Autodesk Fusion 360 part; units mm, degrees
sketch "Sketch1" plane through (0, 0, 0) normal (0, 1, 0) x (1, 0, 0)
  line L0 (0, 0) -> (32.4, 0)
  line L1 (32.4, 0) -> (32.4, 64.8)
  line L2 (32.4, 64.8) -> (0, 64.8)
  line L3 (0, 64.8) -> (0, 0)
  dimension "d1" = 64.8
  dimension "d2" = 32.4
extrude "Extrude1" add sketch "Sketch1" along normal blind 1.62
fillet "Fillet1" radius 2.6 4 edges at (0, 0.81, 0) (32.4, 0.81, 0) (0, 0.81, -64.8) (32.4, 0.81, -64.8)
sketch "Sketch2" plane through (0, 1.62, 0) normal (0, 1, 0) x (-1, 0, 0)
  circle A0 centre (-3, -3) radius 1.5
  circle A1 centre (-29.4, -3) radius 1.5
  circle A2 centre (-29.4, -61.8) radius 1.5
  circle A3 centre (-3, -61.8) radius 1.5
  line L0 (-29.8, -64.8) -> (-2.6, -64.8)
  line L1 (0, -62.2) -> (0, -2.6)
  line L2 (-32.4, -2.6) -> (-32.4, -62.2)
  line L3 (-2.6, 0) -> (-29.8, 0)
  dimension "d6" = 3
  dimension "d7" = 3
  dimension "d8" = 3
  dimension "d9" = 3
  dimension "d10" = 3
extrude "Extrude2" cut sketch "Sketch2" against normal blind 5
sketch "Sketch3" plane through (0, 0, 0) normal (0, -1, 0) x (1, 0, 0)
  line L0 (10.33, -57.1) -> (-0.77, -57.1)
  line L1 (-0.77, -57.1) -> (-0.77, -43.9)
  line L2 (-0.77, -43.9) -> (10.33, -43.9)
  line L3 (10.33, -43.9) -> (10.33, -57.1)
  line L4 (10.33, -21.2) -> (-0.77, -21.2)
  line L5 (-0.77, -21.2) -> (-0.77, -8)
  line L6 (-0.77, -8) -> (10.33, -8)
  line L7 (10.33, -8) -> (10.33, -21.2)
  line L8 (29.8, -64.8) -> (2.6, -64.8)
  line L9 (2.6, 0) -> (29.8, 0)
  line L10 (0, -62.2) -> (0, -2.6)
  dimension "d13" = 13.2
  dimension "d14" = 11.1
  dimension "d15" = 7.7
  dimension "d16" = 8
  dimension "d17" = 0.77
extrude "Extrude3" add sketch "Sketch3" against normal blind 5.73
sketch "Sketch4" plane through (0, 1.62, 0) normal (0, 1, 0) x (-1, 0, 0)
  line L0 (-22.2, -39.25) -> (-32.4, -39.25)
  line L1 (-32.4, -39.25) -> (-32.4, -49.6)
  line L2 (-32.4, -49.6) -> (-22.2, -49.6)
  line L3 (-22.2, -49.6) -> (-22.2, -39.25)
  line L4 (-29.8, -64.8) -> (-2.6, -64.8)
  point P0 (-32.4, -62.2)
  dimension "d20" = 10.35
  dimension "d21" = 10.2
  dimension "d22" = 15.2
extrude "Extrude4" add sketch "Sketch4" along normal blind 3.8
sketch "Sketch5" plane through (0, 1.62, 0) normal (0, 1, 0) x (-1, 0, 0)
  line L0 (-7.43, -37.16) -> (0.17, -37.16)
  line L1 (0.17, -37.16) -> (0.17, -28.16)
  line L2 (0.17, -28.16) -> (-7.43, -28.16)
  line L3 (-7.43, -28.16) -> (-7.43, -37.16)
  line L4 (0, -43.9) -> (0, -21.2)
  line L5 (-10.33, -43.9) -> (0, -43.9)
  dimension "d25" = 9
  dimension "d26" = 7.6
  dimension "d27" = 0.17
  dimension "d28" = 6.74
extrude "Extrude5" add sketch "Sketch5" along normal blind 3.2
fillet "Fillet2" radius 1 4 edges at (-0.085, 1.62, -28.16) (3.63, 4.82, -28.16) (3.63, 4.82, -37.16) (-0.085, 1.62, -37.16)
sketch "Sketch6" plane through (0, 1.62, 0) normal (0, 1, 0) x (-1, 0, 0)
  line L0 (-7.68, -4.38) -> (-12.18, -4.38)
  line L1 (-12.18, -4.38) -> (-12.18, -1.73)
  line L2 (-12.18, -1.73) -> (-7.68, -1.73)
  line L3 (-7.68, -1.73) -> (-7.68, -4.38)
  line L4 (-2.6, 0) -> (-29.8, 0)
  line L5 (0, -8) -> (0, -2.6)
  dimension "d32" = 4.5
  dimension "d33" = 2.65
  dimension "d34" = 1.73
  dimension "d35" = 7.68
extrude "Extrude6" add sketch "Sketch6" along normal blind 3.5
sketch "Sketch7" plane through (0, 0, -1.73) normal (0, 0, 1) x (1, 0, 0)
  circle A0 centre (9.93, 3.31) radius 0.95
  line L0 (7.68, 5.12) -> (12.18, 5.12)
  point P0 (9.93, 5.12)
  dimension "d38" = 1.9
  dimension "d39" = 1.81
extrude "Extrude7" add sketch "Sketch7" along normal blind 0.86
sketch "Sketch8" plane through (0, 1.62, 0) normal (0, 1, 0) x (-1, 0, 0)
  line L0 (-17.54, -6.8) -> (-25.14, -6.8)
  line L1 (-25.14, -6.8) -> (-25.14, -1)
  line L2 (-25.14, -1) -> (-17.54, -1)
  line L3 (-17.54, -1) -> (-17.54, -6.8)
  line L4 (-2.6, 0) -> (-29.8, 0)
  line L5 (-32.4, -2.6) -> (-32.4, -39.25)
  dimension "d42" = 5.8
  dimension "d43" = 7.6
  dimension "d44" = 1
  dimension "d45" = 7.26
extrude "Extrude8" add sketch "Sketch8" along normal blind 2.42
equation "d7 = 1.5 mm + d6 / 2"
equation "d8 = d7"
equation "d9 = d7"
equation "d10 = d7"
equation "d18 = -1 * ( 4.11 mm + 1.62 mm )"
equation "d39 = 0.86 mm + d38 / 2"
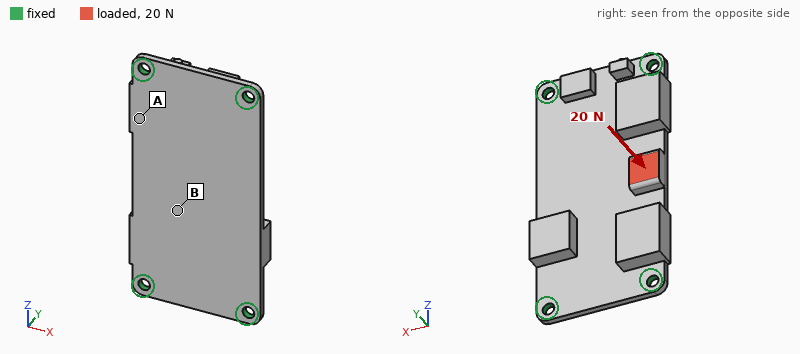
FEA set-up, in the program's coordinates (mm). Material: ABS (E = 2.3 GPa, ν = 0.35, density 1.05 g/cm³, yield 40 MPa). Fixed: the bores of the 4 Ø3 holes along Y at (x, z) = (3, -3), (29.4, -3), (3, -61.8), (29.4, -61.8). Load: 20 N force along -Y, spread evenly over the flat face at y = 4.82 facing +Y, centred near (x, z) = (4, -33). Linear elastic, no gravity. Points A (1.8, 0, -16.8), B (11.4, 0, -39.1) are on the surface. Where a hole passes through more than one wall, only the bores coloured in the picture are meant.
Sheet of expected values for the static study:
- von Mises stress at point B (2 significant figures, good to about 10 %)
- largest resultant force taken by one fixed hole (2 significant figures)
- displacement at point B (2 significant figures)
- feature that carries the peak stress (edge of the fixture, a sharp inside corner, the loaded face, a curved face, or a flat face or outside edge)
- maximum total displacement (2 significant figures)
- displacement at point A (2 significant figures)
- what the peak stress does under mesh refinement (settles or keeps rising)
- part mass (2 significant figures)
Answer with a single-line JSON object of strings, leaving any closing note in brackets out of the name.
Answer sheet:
{"von Mises stress at point B": "5.4 MPa", "largest resultant force taken by one fixed hole": "9.4 N", "displacement at point B": "0.60 mm", "feature that carries the peak stress": "edge of the fixture", "maximum total displacement": "0.81 mm", "displacement at point A": "0.40 mm", "what the peak stress does under mesh refinement": "keeps rising", "part mass": "5.6 g"}
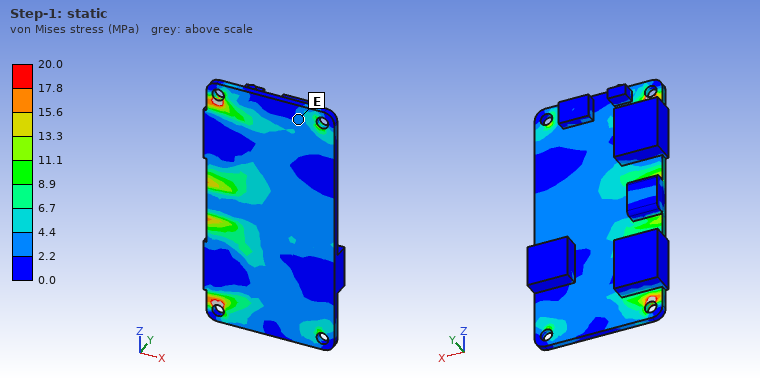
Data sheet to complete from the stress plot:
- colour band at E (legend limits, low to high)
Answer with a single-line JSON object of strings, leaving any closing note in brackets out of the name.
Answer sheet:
{"colour band at E": "2.2 to 4.4 MPa"}
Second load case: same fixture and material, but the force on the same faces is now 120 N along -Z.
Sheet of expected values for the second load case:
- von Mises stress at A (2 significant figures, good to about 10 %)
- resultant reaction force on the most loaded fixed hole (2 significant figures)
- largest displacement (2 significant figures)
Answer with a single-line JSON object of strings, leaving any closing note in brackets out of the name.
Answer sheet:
{"von Mises stress at A": "2.3 MPa", "resultant reaction force on the most loaded fixed hole": "44 N", "largest displacement": "0.43 mm"}
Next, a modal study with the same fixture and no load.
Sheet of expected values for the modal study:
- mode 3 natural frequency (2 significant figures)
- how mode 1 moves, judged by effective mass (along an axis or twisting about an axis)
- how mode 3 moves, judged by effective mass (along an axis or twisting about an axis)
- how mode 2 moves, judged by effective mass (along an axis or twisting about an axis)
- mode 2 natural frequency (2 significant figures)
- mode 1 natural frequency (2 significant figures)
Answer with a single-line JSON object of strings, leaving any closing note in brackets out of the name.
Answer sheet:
{"mode 3 natural frequency": "1800 Hz", "how mode 1 moves, judged by effective mass": "along Y", "how mode 3 moves, judged by effective mass": "twisting about X", "how mode 2 moves, judged by effective mass": "twisting about Z", "mode 2 natural frequency": "1200 Hz", "mode 1 natural frequency": "620 Hz"}
